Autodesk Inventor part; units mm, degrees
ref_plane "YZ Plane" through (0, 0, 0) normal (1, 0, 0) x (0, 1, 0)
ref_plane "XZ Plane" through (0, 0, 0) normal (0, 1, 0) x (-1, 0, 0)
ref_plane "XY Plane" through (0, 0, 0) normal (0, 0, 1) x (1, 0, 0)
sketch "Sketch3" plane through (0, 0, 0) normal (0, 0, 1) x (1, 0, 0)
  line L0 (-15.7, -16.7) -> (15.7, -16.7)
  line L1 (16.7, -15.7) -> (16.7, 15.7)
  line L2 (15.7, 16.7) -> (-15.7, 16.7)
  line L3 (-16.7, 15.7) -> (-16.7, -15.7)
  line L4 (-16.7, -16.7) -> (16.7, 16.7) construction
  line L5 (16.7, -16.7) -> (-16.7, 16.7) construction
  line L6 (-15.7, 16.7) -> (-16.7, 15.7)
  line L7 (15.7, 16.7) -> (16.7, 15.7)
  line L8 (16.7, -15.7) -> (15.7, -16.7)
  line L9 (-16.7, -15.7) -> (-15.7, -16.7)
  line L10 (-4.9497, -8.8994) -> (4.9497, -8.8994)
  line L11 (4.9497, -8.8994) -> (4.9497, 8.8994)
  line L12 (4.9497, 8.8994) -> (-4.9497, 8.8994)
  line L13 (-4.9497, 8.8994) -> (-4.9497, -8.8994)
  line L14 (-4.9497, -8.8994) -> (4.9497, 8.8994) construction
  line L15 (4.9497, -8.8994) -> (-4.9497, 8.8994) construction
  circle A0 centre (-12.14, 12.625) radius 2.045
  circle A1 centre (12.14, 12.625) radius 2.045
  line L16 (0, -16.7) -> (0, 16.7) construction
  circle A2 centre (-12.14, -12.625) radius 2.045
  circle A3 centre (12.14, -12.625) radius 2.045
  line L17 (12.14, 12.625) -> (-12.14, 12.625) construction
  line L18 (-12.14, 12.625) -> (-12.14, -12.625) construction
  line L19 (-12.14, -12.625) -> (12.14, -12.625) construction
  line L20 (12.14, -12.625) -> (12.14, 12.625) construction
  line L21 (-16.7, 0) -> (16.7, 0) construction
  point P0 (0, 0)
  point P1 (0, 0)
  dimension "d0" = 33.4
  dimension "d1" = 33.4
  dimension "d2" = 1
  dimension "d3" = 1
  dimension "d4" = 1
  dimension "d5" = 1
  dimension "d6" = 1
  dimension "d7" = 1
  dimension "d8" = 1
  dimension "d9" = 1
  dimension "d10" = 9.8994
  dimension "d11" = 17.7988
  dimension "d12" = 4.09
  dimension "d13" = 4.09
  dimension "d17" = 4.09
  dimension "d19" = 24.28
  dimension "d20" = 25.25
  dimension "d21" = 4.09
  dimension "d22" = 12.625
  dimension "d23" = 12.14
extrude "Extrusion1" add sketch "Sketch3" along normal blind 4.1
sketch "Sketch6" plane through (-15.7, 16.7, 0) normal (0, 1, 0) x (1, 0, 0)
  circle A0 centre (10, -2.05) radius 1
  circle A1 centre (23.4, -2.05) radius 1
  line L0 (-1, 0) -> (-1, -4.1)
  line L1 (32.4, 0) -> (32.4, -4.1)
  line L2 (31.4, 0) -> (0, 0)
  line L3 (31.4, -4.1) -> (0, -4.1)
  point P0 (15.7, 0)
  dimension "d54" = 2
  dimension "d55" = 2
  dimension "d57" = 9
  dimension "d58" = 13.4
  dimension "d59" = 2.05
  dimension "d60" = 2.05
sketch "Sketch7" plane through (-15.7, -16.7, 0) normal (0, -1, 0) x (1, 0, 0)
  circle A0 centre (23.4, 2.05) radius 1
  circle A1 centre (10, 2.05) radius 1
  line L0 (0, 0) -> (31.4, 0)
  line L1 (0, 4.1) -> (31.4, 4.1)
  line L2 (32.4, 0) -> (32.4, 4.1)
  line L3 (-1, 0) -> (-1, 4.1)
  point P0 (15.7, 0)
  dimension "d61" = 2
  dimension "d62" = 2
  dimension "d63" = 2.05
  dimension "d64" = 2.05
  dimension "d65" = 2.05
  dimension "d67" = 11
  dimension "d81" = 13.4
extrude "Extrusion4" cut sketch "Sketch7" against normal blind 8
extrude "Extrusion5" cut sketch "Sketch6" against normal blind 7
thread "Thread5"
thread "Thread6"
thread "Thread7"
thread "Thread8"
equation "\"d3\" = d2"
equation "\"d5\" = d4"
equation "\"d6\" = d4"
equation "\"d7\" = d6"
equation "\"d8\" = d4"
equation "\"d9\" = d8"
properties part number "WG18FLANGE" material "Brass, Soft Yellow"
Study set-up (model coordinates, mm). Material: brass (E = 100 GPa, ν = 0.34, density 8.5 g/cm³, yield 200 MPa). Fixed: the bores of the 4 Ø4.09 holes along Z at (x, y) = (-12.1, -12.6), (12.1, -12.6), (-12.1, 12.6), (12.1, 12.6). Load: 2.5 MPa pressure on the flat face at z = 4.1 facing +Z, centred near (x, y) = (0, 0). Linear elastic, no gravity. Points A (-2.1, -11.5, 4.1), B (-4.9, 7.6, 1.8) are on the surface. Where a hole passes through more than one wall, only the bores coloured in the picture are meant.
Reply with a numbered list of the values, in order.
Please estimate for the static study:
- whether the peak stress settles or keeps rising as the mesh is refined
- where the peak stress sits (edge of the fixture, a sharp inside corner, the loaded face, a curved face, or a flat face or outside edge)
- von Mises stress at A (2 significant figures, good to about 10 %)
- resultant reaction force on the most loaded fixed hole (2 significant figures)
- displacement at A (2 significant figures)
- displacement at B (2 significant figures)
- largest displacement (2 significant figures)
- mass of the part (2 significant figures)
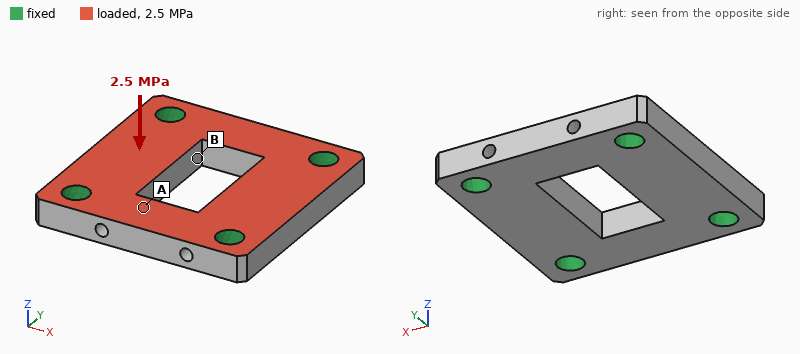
1. keeps rising
2. edge of the fixture
3. 15 MPa
4. 560 N
5. 4.8 µm
6. 4.9 µm
7. 7.9 µm
8. 30 g
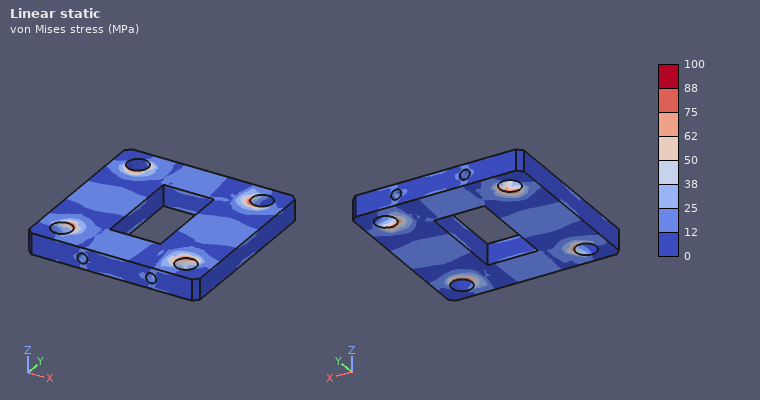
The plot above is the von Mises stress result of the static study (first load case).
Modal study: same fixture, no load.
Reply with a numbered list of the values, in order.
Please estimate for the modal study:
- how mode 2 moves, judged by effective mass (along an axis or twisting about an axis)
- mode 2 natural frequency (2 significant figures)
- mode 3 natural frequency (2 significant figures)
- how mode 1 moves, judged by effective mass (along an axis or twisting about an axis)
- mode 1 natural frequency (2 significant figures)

1. twisting about Y
2. 22 kHz
3. 24 kHz
4. along Z
5. 20 kHz
